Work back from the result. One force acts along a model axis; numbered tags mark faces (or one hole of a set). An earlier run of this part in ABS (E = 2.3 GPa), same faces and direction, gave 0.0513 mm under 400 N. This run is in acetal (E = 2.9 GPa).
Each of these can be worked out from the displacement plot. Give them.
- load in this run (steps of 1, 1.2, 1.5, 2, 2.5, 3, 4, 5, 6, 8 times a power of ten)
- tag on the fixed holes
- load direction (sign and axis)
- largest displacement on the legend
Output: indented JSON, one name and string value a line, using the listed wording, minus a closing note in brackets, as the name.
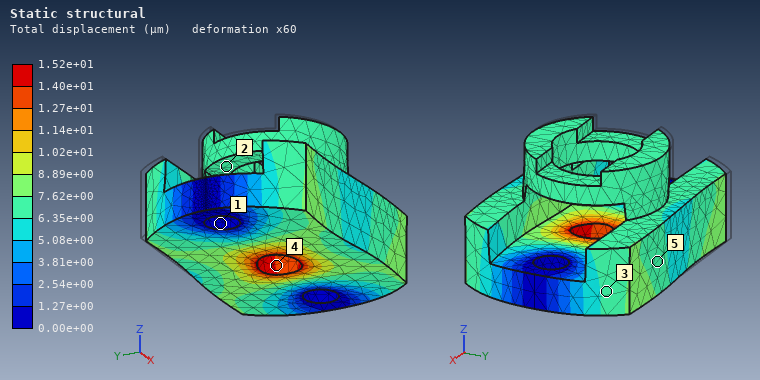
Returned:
{
  "load in this run": "150 N",
  "tag on the fixed holes": "1",
  "load direction": "+X",
  "largest displacement on the legend": "1.52e+01 µm"
}
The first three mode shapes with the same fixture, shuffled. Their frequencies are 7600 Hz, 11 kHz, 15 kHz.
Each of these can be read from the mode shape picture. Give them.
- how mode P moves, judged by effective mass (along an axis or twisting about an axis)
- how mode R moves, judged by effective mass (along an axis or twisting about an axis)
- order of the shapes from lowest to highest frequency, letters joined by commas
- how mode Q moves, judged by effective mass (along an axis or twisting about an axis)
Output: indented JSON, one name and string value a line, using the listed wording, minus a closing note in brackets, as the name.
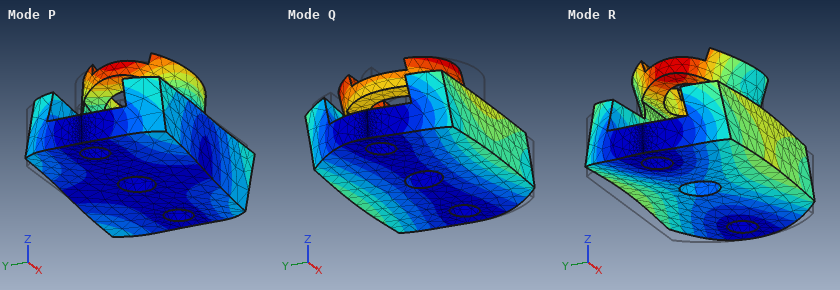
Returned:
{
  "how mode P moves, judged by effective mass": "along X",
  "how mode R moves, judged by effective mass": "along Z",
  "order of the shapes from lowest to highest frequency, letters joined by commas": "Q, R, P",
  "how mode Q moves, judged by effective mass": "along Y"
}
